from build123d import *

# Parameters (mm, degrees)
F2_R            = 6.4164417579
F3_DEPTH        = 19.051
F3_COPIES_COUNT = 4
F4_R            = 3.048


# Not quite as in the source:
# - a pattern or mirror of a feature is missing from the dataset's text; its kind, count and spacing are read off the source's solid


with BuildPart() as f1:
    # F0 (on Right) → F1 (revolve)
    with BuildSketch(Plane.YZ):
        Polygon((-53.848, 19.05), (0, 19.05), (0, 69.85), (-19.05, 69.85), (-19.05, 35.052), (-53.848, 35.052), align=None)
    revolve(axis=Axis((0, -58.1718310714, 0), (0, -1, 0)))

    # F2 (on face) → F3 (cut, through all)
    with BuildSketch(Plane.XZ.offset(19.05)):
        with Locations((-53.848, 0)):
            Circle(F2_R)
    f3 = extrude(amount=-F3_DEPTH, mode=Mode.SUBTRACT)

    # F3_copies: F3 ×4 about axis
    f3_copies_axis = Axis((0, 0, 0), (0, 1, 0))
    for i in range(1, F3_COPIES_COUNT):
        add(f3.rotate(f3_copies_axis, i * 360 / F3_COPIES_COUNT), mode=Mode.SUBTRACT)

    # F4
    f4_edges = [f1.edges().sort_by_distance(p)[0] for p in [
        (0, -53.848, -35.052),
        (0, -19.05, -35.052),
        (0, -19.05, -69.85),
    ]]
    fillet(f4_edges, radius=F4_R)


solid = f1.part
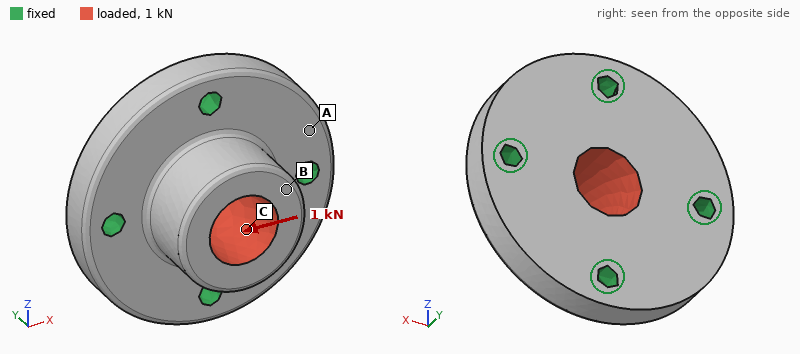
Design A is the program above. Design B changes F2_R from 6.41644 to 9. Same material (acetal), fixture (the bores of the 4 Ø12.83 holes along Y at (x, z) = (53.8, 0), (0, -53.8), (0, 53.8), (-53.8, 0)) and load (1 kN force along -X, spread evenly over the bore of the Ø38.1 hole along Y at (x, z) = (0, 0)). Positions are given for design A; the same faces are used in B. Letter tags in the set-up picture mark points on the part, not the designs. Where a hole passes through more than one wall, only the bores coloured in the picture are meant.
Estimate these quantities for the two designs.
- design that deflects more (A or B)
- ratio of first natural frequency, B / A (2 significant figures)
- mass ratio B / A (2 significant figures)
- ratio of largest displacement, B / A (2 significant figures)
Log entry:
A
1.1
0.97
0.90
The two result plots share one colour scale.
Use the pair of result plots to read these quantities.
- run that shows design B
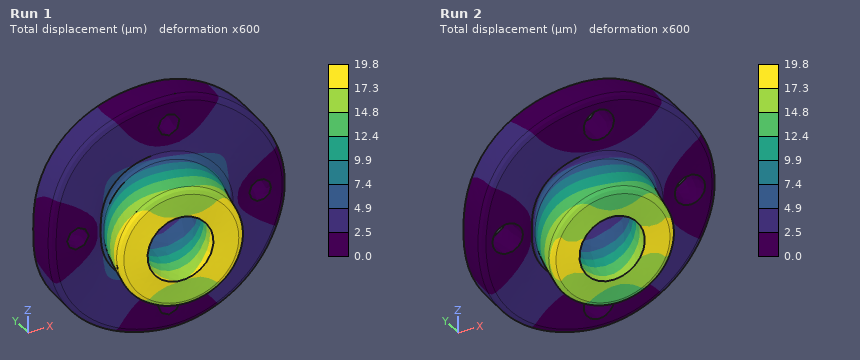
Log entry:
Run 2
